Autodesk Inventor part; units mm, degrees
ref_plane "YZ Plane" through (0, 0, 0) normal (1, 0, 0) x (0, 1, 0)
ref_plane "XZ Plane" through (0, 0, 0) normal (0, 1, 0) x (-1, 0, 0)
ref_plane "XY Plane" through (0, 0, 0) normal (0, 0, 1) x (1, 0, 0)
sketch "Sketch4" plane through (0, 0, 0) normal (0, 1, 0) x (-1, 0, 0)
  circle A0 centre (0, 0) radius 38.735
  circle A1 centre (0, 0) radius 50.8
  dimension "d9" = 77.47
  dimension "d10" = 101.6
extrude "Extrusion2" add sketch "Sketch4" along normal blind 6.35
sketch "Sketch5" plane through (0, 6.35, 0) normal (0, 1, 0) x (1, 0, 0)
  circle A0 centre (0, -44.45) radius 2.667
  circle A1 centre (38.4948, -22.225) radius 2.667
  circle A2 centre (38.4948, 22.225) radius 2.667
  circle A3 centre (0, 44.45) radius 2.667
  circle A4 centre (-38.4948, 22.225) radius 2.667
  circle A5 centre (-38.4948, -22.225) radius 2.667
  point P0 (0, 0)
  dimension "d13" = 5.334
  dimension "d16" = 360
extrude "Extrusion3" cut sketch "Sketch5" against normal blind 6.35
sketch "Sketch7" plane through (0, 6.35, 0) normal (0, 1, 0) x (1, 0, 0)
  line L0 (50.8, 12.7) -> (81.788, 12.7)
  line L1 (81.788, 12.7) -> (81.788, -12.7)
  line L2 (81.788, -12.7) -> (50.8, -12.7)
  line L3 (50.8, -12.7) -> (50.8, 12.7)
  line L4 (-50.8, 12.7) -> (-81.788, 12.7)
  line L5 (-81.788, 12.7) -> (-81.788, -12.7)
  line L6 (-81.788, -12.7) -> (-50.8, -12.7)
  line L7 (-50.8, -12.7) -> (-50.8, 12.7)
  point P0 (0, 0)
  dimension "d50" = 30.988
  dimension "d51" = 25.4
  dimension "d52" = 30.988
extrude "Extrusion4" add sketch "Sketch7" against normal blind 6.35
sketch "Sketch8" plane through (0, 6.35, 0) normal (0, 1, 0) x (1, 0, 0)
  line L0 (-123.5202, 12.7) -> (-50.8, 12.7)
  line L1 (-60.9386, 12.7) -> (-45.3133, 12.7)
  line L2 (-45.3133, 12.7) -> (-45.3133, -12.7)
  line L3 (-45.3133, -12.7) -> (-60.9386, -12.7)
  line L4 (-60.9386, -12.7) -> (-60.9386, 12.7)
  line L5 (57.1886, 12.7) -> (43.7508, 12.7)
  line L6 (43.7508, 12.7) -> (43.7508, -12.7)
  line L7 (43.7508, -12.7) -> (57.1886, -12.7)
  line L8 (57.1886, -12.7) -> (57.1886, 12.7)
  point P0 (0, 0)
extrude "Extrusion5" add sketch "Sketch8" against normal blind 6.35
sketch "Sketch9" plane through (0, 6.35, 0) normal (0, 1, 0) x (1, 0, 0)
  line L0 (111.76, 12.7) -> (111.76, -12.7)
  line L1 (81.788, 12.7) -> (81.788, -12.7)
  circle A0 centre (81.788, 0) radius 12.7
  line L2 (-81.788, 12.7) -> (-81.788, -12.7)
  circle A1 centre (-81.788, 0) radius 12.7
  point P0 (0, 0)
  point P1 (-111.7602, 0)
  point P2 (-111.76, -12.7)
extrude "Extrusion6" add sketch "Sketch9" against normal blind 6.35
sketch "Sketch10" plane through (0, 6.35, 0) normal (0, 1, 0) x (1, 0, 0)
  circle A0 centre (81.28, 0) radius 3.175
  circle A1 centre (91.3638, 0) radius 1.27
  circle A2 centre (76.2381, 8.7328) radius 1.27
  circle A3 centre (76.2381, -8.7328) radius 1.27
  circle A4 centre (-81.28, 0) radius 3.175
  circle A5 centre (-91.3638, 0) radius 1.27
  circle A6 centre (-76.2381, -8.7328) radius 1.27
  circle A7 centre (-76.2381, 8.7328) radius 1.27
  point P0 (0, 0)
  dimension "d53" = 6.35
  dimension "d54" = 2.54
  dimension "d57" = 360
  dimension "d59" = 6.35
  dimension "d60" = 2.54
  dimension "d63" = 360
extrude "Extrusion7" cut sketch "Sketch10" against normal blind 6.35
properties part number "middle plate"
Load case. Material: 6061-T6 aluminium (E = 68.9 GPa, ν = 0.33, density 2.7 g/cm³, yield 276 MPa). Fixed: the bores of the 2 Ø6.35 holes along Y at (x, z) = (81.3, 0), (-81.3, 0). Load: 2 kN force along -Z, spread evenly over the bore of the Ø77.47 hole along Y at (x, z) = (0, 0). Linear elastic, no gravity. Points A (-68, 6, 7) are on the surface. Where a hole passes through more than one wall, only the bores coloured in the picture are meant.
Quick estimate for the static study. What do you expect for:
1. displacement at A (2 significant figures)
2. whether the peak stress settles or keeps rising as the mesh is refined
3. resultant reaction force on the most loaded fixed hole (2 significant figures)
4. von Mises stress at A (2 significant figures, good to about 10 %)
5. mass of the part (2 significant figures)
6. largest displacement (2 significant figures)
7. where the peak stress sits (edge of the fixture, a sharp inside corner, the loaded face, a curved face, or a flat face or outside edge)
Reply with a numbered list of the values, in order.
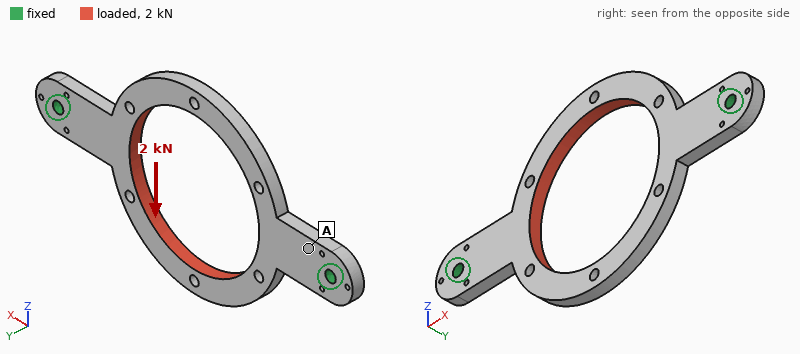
1. 17 µm
2. keeps rising
3. 1.0 kN
4. 11 MPa
5. 90 g
6. 51 µm
7. edge of the fixture
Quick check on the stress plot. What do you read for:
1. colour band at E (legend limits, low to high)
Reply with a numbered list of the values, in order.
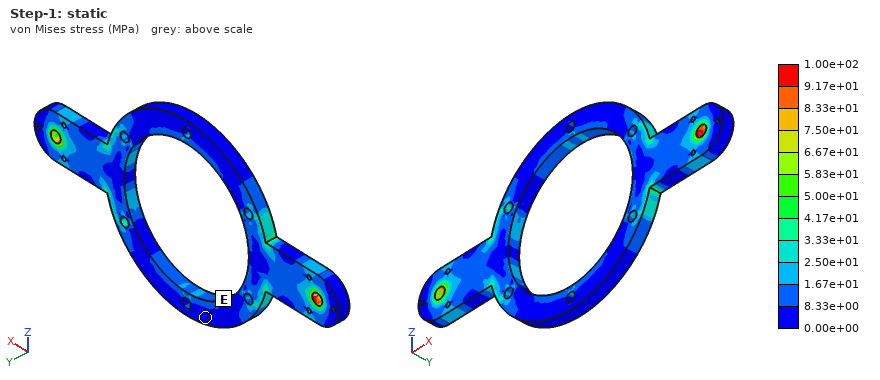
1. 0.00e+00 to 8.33e+00 MPa
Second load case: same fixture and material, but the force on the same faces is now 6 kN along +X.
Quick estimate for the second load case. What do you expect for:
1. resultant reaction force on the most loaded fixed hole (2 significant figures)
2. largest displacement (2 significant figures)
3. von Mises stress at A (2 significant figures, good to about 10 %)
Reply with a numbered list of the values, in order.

1. 3.0 kN
2. 74 µm
3. 19 MPa
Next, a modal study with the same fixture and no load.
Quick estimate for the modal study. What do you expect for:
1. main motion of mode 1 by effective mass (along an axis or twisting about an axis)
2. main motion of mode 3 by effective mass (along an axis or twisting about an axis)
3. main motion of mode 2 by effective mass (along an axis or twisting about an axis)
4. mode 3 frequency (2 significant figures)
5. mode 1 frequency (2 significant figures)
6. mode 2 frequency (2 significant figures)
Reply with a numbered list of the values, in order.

1. twisting about X
2. twisting about Z
3. along Y
4. 2400 Hz
5. 900 Hz
6. 960 Hz
